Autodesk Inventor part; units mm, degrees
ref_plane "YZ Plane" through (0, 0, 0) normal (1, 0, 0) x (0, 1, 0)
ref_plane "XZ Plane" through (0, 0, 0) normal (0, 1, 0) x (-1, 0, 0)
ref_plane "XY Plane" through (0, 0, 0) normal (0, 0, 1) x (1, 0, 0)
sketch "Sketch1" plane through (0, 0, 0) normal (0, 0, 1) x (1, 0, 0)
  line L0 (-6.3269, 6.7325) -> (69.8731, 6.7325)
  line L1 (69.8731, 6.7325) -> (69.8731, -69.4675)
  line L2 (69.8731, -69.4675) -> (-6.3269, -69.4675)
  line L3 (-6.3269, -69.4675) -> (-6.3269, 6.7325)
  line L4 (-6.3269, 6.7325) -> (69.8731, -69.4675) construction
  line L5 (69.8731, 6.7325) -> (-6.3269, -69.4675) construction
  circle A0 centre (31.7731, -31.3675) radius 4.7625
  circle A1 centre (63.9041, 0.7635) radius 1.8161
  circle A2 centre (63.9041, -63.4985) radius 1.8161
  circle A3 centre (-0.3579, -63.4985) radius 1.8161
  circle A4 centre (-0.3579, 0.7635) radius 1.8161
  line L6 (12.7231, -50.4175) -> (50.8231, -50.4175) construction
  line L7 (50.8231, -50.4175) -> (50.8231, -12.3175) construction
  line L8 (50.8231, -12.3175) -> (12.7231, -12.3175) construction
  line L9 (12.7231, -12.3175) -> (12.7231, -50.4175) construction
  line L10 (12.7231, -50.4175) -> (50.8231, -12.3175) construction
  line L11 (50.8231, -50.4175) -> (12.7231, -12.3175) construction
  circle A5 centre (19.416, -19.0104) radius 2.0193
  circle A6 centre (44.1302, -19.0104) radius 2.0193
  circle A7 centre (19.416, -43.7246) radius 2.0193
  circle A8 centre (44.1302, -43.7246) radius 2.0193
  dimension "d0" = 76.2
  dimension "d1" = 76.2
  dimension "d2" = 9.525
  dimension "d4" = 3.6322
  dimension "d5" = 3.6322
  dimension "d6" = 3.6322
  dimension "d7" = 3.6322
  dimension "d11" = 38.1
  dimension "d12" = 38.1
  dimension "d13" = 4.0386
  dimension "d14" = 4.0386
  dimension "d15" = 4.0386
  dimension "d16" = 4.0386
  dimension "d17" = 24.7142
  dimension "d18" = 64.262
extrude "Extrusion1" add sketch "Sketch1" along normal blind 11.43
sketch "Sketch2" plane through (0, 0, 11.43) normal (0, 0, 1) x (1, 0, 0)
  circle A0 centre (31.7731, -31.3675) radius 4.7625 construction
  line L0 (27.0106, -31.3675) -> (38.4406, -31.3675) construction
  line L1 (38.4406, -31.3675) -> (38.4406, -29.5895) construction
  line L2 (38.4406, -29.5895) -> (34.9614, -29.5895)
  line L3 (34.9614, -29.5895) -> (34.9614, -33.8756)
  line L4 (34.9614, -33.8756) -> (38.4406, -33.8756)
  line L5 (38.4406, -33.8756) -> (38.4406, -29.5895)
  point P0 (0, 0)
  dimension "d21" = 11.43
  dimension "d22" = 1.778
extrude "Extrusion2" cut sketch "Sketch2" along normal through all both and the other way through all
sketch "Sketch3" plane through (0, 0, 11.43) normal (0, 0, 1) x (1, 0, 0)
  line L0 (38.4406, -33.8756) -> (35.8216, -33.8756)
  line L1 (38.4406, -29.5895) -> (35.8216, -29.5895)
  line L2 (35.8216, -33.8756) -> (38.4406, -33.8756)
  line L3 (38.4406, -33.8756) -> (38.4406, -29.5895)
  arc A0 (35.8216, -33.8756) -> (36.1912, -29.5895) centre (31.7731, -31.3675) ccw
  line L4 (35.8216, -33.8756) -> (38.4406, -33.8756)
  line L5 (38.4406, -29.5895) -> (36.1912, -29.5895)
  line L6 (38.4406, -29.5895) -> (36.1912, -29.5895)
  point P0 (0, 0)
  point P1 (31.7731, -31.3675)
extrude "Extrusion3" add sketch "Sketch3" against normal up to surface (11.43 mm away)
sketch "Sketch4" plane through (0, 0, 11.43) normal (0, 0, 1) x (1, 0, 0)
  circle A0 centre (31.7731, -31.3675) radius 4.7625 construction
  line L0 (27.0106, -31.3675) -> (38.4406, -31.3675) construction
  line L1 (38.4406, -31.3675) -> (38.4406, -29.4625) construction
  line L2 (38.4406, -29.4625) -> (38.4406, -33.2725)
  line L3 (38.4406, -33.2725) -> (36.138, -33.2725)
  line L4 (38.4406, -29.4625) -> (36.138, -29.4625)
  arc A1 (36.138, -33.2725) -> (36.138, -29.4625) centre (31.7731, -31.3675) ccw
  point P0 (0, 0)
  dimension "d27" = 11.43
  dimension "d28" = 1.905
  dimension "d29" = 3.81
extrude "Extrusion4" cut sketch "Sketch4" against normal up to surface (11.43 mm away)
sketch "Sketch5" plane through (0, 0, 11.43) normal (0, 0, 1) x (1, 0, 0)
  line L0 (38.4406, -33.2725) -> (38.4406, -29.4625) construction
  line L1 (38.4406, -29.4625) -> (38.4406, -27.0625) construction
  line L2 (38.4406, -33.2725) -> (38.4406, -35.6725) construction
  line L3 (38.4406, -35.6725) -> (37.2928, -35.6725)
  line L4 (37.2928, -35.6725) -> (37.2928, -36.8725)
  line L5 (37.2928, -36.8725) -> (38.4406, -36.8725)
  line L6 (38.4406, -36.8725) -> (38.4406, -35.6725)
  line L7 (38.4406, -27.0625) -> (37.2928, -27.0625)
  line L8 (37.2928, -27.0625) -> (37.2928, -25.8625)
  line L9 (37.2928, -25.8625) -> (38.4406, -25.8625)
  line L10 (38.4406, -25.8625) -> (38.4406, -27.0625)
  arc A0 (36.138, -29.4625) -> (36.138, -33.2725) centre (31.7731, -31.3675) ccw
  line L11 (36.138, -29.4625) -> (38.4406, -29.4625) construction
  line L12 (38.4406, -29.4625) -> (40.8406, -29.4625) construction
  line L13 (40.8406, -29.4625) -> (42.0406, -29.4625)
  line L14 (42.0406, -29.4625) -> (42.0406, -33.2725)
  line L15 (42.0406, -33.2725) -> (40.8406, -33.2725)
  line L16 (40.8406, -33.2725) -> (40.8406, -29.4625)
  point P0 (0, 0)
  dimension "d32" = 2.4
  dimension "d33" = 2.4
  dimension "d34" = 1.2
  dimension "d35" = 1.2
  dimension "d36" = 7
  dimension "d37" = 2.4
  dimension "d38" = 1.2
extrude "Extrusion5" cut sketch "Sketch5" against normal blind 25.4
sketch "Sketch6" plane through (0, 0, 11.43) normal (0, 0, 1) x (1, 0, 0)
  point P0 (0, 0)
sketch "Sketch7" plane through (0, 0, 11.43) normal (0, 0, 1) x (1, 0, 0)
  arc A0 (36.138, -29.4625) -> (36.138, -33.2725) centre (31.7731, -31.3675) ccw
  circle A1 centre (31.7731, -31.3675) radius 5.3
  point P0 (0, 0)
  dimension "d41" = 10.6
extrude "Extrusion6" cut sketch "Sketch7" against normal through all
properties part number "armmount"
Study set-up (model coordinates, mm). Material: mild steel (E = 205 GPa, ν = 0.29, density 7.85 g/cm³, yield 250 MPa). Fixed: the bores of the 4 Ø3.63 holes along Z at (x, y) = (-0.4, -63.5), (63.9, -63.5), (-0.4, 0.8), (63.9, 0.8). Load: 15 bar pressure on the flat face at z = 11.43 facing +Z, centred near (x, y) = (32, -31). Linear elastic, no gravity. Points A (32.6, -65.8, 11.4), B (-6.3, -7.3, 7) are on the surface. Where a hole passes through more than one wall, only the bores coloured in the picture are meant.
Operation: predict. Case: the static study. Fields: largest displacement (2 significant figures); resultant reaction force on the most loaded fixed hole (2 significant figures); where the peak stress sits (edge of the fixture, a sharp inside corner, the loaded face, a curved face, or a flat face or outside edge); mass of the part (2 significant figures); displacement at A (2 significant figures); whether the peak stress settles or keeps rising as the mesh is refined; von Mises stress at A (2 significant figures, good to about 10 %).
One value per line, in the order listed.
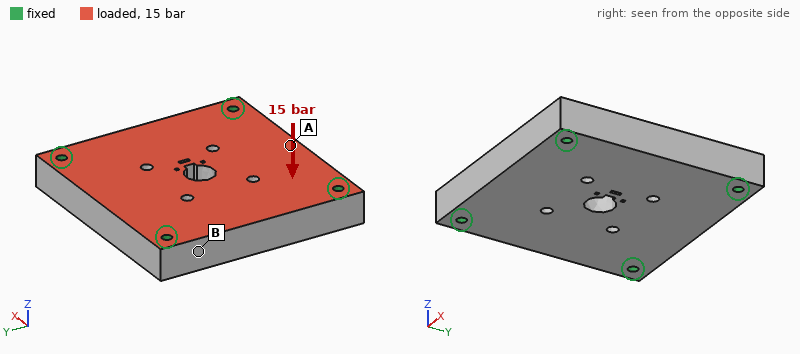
11 µm
2.1 kN
edge of the fixture
500 g
6.0 µm
keeps rising
18 MPa
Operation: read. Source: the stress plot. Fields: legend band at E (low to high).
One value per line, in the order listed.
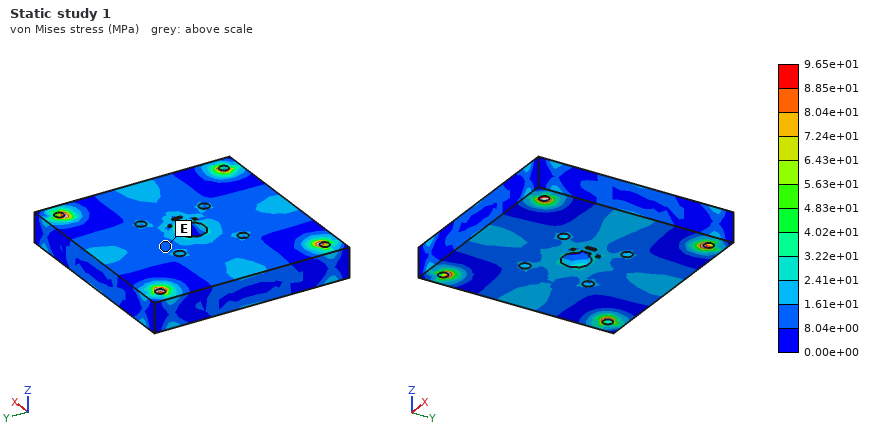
8.04e+00 to 1.61e+01 MPa
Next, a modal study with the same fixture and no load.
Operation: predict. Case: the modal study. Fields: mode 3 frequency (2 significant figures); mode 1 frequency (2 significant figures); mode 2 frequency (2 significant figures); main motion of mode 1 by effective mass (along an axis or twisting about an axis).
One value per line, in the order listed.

12 kHz
7500 Hz
12 kHz
along Z
